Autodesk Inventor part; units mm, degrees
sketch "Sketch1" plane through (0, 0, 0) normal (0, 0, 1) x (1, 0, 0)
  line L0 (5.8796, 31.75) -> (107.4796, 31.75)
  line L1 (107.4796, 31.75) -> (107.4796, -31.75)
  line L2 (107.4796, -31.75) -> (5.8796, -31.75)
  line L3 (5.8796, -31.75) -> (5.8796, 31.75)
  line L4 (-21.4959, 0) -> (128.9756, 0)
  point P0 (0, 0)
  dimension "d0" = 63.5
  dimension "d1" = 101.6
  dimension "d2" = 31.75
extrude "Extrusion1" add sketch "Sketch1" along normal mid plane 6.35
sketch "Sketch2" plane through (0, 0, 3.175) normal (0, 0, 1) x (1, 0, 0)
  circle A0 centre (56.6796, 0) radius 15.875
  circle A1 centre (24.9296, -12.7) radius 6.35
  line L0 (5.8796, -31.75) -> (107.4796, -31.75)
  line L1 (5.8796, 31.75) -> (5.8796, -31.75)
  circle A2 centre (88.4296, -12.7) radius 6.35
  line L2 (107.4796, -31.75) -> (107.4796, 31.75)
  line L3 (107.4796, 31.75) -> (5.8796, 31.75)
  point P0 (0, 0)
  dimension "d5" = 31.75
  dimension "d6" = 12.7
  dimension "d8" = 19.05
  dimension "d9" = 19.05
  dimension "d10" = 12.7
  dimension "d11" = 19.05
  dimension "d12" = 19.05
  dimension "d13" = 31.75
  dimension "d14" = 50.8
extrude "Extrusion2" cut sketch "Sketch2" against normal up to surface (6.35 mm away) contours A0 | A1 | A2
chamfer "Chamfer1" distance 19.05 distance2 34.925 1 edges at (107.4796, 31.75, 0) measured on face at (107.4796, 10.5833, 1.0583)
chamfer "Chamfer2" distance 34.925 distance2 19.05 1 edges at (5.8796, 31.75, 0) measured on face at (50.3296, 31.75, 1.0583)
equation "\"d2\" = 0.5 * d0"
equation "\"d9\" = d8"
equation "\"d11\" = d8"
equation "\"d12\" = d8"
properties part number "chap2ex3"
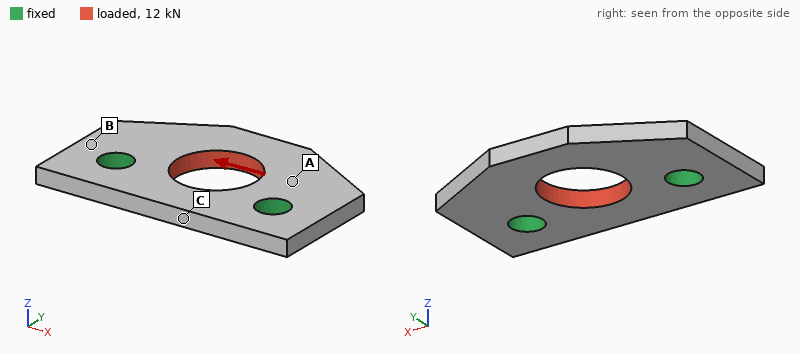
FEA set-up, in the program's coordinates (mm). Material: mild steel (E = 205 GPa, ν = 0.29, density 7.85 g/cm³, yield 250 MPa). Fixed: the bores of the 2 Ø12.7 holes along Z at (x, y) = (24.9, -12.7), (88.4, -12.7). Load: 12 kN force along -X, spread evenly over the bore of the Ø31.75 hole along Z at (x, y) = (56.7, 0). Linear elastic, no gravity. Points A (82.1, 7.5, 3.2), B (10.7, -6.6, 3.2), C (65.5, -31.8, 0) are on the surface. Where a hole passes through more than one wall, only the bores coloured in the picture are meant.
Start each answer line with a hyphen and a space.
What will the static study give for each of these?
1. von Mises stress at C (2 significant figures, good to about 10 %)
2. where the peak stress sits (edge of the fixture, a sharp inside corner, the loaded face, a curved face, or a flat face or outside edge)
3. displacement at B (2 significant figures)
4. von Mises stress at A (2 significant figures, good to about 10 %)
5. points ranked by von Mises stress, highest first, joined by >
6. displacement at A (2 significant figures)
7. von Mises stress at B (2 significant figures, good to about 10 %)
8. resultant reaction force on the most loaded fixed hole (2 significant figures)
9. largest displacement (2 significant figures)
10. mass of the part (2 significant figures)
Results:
- 8.2 MPa
- edge of the fixture
- 2.6 µm
- 31 MPa
- A > B > C
- 6.4 µm
- 17 MPa
- 6.1 kN
- 11 µm
- 240 g
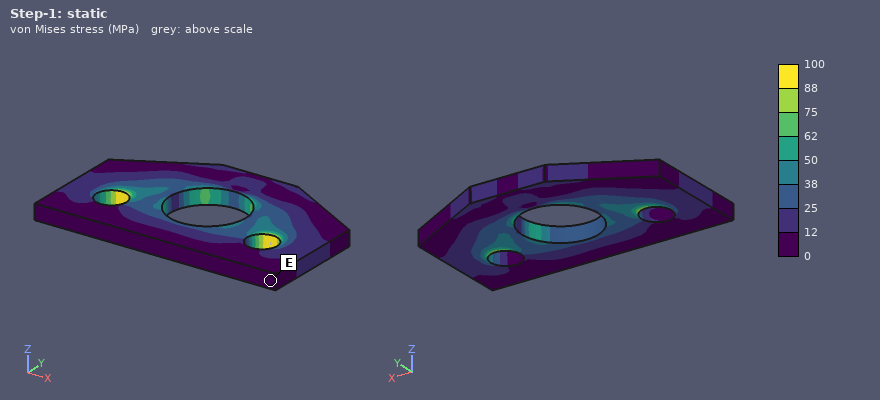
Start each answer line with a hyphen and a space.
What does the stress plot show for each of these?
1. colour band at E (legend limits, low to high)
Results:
- 0 to 12 MPa
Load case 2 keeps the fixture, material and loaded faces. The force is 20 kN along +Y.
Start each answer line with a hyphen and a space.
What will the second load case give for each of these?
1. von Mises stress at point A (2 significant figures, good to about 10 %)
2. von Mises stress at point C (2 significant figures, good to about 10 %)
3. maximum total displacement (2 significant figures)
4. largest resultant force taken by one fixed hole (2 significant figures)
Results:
- 46 MPa
- 49 MPa
- 14 µm
- 10 kN
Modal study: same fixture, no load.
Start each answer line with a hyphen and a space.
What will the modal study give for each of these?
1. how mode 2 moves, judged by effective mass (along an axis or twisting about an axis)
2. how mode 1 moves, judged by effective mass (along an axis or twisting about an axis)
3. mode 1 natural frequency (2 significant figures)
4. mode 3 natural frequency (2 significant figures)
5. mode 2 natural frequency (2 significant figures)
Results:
- twisting about Y
- along Z
- 3100 Hz
- 9100 Hz
- 6200 Hz
